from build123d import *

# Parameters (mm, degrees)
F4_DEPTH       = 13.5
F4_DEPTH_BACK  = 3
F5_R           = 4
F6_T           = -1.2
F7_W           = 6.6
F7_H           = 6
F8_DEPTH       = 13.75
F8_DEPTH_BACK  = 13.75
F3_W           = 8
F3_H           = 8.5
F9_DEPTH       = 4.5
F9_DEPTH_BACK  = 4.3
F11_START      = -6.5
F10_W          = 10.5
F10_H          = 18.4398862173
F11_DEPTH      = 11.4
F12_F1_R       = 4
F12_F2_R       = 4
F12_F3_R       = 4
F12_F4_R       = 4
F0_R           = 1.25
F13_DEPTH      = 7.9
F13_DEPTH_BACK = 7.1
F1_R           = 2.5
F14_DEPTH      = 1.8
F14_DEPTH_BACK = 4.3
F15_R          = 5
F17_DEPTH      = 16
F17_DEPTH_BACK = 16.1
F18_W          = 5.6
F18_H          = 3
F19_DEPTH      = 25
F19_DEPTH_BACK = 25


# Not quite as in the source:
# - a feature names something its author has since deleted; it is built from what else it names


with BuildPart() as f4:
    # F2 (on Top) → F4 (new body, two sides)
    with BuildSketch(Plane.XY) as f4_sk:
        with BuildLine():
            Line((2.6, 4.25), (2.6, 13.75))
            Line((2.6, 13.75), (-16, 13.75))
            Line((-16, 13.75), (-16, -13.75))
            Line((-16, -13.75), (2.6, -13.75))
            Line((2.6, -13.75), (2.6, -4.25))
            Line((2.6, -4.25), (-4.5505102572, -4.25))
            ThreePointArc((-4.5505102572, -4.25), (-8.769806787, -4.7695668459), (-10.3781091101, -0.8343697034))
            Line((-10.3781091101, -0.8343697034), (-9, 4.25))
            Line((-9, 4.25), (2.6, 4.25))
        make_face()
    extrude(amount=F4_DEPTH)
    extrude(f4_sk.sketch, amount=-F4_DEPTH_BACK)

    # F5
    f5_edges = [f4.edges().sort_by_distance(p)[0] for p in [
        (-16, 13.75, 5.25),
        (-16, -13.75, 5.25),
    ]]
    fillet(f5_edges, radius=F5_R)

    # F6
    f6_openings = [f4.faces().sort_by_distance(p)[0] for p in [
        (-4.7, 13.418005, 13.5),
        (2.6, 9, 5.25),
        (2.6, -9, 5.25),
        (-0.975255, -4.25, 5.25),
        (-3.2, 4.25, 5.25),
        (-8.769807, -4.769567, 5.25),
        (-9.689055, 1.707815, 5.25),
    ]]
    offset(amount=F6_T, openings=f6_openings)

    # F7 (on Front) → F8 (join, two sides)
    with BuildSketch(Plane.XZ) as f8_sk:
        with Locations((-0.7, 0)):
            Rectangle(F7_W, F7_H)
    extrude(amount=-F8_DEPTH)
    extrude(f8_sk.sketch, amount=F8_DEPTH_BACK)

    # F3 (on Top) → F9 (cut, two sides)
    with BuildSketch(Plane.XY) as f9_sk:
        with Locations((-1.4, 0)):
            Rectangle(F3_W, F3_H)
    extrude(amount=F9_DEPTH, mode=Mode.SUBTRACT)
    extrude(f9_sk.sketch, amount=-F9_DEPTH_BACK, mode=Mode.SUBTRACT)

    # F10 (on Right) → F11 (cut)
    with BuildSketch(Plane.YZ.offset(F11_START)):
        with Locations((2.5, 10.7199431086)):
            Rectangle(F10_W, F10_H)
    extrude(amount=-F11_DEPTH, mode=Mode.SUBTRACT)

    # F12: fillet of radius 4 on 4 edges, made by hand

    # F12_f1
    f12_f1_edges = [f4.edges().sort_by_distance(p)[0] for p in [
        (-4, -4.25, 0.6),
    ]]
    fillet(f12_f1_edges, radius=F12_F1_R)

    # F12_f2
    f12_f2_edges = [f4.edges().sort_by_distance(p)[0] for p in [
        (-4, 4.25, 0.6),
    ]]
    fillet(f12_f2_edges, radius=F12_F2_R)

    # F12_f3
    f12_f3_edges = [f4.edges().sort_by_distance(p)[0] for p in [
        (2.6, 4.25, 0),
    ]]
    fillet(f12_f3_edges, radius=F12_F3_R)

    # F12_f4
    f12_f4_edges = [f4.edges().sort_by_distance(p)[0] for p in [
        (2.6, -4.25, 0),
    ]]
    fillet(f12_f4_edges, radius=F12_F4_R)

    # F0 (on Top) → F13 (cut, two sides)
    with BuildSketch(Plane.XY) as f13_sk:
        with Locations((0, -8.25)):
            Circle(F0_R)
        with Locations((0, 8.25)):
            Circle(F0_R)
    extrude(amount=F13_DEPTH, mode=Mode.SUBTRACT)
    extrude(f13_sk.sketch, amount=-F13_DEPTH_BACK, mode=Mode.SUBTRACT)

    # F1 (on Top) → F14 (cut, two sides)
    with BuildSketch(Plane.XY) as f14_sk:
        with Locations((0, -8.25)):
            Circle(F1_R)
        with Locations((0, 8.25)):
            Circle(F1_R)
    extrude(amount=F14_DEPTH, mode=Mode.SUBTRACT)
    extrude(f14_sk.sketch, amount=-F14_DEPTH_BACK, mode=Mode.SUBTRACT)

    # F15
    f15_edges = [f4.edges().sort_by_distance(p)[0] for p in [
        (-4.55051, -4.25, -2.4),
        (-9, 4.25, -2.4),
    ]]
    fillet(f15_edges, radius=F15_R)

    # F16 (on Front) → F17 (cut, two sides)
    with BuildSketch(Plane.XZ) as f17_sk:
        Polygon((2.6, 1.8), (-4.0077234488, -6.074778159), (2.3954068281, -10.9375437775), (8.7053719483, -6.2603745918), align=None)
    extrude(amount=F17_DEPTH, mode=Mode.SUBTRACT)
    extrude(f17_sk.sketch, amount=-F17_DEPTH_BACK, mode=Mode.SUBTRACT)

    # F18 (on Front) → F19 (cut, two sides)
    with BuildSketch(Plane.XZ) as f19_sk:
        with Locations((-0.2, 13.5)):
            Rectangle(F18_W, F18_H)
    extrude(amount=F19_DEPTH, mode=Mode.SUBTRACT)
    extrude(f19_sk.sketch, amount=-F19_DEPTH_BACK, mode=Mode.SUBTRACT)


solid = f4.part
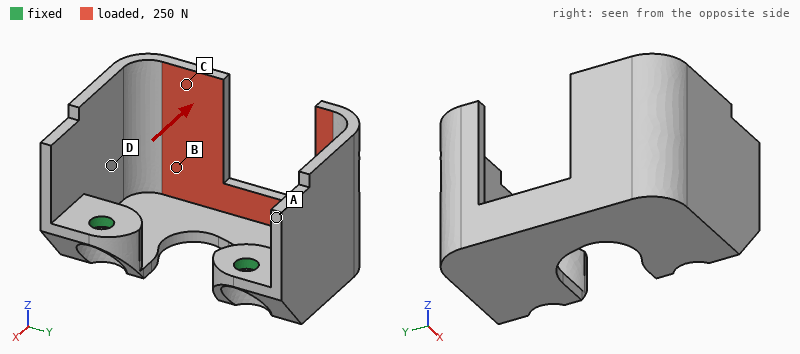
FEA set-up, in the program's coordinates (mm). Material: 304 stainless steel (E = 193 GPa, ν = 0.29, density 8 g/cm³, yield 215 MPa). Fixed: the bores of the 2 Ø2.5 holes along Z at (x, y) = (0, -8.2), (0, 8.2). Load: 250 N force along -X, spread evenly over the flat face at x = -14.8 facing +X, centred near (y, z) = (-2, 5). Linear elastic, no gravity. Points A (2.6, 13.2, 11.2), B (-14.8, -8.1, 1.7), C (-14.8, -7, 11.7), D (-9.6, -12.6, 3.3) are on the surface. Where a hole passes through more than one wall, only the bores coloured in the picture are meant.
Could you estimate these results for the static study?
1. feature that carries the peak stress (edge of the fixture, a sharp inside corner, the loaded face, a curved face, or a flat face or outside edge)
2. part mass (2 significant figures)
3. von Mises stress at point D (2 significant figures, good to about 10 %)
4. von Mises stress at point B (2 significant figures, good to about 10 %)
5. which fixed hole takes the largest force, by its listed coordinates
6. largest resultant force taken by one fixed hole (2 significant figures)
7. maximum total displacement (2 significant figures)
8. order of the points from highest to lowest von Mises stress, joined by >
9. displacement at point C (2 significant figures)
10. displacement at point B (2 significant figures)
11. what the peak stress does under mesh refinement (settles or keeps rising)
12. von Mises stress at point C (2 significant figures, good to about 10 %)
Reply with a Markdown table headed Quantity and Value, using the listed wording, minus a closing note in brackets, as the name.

| Quantity | Value |
|---|---|
| feature that carries the peak stress | edge of the fixture |
| part mass | 12 g |
| von Mises stress at point D | 37 MPa |
| von Mises stress at point B | 82 MPa |
| which fixed hole takes the largest force, by its listed coordinates | (0, -8.2) |
| largest resultant force taken by one fixed hole | 150 N |
| maximum total displacement | 0.11 mm |
| order of the points from highest to lowest von Mises stress, joined by > | B > C > D > A |
| displacement at point C | 0.066 mm |
| displacement at point B | 0.026 mm |
| what the peak stress does under mesh refinement | keeps rising |
| von Mises stress at point C | 60 MPa |
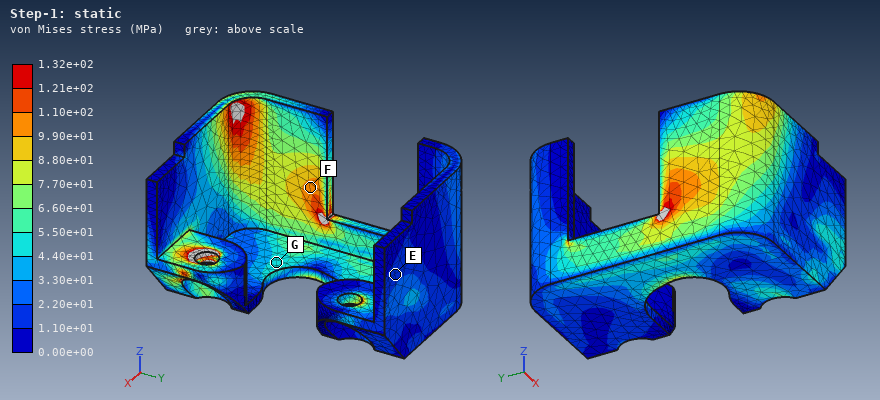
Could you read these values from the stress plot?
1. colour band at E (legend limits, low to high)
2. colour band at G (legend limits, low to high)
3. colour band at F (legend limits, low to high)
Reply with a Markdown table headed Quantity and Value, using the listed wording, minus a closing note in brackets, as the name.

| Quantity | Value |
|---|---|
| colour band at E | 1.10e+01 to 2.20e+01 MPa |
| colour band at G | 4.40e+01 to 5.50e+01 MPa |
| colour band at F | 9.90e+01 to 1.10e+02 MPa |
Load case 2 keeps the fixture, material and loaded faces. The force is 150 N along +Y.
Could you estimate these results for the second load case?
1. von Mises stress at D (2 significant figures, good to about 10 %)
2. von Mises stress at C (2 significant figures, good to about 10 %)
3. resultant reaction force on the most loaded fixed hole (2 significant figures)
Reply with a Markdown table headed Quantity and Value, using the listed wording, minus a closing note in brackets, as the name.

| Quantity | Value |
|---|---|
| von Mises stress at D | 18 MPa |
| von Mises stress at C | 19 MPa |
| resultant reaction force on the most loaded fixed hole | 100 N |
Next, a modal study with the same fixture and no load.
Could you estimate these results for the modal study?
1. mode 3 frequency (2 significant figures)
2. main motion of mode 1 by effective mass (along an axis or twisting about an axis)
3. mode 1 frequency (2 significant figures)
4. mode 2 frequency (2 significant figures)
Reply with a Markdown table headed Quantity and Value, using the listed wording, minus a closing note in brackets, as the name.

| Quantity | Value |
|---|---|
| mode 3 frequency | 7500 Hz |
| main motion of mode 1 by effective mass | along Z |
| mode 1 frequency | 3500 Hz |
| mode 2 frequency | 3900 Hz |
